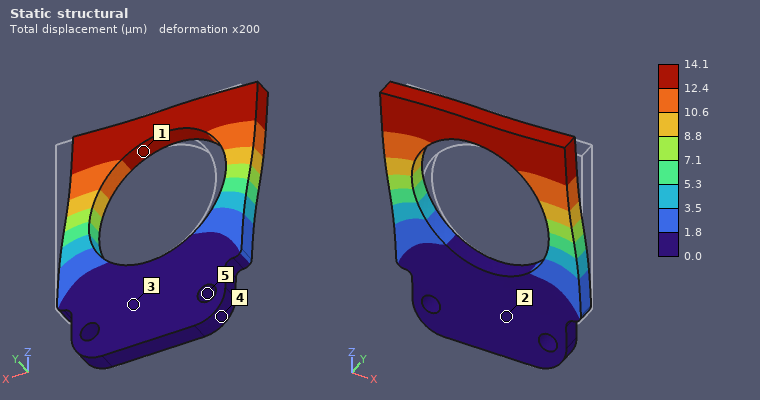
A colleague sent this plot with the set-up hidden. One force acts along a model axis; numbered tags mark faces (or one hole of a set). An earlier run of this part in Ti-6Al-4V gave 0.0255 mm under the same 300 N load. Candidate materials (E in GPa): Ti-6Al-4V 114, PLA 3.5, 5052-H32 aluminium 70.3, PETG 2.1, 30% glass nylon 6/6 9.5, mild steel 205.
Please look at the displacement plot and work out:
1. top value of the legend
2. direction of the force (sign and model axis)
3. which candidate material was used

14.1 µm
-X
mild steel
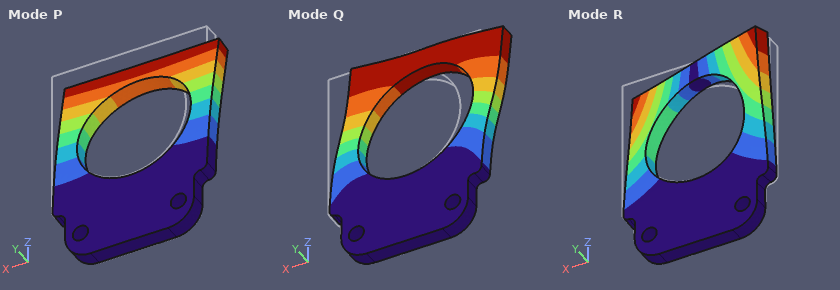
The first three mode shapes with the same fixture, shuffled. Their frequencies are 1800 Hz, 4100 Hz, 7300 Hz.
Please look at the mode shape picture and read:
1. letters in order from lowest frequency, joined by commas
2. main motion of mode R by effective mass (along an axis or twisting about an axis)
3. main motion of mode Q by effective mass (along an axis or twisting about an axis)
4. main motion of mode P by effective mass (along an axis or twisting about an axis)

P, R, Q
twisting about Z
along X
along Y
